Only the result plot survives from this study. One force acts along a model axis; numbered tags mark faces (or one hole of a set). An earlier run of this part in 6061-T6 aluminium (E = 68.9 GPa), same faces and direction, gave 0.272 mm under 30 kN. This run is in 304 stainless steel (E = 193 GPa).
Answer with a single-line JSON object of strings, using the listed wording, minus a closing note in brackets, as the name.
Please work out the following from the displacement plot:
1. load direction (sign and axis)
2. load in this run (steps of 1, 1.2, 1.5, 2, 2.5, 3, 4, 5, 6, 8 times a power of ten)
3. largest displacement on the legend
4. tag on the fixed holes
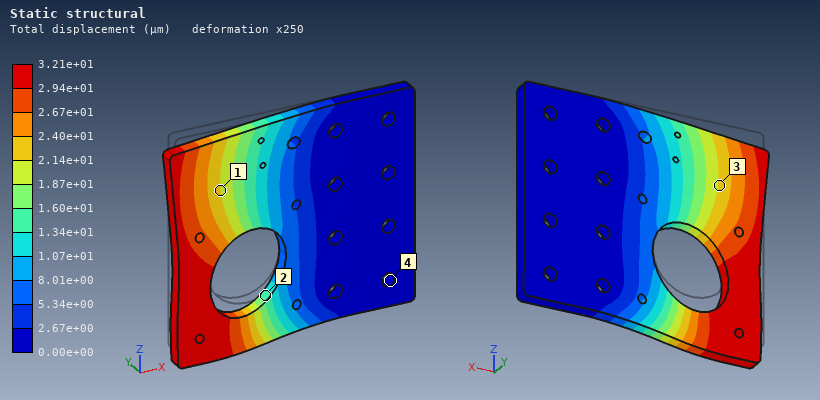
{"load direction": "-Z", "load in this run": "10 kN", "largest displacement on the legend": "3.21e+01 µm", "tag on the fixed holes": "4"}
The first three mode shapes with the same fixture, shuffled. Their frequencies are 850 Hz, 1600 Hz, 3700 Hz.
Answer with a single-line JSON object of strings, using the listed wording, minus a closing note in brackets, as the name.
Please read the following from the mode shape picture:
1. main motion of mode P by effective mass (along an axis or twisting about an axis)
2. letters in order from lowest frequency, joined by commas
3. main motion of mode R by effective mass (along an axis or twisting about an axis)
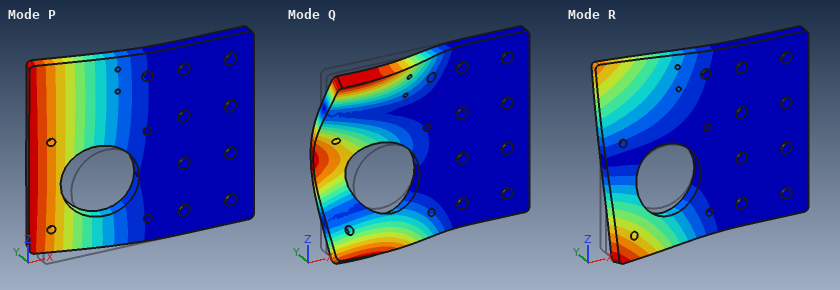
{"main motion of mode P by effective mass": "along Y", "letters in order from lowest frequency, joined by commas": "P, R, Q", "main motion of mode R by effective mass": "twisting about X"}
